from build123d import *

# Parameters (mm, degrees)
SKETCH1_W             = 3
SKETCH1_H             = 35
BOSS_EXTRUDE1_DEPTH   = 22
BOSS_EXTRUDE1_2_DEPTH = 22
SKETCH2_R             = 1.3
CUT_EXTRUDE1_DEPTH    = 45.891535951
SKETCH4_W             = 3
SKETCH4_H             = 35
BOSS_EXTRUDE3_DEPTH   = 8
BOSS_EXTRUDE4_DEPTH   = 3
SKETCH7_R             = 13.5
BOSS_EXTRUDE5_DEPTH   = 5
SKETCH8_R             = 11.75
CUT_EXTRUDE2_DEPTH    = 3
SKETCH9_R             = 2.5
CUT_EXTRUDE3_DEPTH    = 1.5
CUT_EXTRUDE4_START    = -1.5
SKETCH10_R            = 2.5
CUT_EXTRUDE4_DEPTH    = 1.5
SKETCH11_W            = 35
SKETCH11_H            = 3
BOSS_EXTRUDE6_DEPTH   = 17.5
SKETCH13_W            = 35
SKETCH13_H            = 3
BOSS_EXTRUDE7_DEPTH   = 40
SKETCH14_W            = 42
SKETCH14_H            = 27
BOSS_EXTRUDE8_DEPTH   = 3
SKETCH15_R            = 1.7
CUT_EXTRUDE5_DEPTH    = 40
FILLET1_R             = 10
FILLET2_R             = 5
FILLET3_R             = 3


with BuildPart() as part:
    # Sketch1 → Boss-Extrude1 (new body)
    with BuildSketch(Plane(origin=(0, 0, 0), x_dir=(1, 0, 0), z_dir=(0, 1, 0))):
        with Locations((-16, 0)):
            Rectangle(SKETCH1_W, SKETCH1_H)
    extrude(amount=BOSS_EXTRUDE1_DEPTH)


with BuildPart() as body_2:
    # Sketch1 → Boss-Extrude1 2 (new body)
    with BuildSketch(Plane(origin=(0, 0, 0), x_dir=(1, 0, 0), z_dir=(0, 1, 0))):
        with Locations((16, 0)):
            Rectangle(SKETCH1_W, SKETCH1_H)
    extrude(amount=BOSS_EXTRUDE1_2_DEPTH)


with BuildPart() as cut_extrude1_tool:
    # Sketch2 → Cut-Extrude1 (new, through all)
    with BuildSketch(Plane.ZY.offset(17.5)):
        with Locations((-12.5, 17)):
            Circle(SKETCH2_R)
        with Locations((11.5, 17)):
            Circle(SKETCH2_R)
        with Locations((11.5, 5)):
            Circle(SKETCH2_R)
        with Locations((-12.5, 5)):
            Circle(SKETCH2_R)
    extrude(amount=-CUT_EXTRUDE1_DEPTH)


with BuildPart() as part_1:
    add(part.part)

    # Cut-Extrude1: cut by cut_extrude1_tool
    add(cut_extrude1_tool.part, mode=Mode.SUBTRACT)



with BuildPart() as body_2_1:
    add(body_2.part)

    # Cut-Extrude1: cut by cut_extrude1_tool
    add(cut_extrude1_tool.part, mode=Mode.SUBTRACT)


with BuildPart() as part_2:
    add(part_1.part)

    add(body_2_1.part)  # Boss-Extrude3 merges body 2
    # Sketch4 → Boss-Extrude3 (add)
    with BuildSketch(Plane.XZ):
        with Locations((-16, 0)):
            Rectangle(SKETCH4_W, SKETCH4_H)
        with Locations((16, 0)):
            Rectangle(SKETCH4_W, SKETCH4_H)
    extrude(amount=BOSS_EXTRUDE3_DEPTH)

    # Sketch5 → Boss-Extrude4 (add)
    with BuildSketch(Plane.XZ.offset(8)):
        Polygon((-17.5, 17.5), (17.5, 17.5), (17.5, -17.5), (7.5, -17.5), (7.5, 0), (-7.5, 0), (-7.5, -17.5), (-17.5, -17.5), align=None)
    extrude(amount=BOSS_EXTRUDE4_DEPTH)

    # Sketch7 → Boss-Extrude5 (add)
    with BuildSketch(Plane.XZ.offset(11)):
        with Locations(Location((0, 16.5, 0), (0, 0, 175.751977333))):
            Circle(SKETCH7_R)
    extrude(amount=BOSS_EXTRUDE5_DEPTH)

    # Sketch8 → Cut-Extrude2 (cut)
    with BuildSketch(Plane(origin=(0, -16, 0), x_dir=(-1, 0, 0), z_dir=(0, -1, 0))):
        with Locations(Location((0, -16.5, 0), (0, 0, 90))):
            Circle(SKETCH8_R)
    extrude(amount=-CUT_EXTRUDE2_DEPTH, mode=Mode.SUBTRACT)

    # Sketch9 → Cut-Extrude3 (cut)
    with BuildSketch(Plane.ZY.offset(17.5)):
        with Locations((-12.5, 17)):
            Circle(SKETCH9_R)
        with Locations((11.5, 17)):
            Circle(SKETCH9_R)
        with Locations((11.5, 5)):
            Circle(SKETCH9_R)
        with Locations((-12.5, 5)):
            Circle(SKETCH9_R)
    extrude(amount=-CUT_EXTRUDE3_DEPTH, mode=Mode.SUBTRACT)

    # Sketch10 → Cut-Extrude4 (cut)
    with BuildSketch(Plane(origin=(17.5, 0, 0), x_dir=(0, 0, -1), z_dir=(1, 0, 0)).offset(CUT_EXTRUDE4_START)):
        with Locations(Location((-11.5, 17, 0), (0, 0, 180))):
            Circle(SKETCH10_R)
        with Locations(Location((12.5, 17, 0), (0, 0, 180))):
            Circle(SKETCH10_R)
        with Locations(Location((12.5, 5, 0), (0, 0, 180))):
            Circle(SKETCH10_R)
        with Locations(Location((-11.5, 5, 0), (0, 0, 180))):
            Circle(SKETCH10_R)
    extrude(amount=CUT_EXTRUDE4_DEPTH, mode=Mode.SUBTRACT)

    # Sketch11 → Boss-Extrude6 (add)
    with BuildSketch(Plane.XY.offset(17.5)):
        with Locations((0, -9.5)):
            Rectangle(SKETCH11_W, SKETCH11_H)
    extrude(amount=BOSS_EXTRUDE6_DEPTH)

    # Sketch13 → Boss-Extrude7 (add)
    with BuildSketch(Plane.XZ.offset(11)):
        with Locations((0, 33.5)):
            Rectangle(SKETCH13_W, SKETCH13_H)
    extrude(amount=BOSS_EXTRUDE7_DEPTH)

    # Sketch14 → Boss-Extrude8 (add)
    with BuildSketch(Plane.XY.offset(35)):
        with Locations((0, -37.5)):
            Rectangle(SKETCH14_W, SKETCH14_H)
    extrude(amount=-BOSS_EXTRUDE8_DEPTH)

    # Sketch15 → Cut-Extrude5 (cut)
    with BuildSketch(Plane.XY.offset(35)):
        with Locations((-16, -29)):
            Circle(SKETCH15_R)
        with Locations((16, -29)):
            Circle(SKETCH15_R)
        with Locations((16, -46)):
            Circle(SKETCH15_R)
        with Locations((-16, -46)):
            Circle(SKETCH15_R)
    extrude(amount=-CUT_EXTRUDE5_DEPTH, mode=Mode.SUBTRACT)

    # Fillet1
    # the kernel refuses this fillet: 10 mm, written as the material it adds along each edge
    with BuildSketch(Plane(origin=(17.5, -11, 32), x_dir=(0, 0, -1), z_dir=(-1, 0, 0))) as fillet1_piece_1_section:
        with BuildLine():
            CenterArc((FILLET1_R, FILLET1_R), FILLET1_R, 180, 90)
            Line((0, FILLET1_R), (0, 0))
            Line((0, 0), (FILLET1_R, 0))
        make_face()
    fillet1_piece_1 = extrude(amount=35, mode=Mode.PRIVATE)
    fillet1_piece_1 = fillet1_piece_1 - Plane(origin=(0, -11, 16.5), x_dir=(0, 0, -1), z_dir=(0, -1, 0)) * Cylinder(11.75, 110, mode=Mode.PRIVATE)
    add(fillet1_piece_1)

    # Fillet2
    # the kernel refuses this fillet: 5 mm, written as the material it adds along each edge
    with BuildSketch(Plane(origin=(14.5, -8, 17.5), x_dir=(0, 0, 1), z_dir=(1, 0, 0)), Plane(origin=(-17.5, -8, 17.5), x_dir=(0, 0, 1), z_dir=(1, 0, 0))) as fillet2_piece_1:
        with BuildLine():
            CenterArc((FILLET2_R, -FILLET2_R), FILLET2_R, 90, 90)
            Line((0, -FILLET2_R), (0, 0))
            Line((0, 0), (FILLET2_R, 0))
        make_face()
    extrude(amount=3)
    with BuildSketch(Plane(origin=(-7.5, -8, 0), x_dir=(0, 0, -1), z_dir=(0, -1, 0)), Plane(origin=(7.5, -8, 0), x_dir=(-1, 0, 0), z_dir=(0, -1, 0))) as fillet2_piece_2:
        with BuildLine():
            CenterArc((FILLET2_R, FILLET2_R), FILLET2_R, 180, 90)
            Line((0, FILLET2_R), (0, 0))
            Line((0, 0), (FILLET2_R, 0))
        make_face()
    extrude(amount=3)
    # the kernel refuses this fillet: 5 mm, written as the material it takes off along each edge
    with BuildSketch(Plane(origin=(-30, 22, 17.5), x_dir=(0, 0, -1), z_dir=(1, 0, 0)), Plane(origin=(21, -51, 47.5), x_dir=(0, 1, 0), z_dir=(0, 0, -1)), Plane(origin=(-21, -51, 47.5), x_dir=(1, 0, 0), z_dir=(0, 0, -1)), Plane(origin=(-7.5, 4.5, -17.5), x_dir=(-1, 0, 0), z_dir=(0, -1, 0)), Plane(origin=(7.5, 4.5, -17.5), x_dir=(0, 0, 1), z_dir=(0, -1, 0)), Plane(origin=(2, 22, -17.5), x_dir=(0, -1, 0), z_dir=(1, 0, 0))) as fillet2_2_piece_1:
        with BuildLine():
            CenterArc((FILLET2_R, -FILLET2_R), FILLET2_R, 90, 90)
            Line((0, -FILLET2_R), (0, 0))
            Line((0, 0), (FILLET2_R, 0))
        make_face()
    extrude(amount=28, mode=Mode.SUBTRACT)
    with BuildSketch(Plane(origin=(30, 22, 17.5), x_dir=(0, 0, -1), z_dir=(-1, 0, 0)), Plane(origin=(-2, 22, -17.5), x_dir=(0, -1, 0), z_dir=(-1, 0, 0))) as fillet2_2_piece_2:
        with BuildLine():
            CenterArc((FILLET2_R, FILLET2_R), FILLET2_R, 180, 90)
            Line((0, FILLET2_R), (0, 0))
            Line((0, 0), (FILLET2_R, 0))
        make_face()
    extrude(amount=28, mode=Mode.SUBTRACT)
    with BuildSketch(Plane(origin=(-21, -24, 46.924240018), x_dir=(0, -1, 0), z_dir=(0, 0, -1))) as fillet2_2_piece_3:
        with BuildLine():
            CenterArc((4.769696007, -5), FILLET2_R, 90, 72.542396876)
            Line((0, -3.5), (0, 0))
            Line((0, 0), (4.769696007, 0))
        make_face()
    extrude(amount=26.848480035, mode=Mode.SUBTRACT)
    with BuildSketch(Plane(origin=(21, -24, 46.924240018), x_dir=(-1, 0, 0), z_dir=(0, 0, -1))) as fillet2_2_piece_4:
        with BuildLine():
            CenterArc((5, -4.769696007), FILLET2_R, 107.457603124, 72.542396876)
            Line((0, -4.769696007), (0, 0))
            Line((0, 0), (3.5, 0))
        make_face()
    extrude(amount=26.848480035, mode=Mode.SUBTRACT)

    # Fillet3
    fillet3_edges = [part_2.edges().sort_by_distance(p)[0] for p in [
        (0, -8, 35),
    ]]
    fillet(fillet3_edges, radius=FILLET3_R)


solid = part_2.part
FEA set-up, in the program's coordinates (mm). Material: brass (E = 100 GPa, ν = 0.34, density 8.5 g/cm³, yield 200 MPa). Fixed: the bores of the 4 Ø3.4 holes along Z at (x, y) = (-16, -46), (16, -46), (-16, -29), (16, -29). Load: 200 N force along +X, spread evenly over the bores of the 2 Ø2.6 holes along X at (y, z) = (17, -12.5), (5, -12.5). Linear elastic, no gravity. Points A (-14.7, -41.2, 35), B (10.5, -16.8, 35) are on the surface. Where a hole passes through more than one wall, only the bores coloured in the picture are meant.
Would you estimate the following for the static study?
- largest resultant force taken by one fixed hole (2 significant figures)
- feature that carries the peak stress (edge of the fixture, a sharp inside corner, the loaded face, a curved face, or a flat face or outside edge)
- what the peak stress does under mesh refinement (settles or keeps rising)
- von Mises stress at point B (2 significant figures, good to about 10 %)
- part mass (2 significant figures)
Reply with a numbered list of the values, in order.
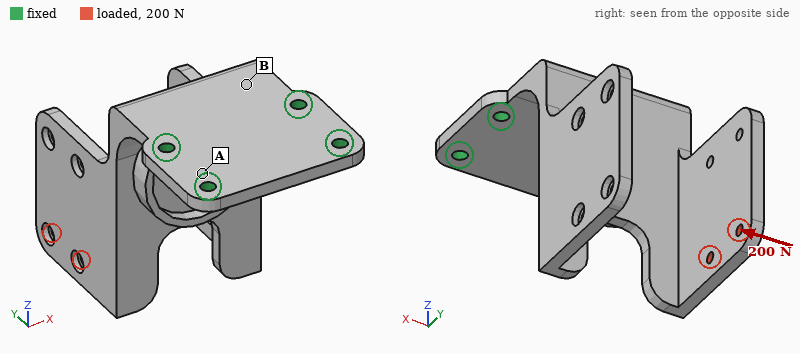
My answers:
1. 410 N
2. edge of the fixture
3. keeps rising
4. 38 MPa
5. 150 g
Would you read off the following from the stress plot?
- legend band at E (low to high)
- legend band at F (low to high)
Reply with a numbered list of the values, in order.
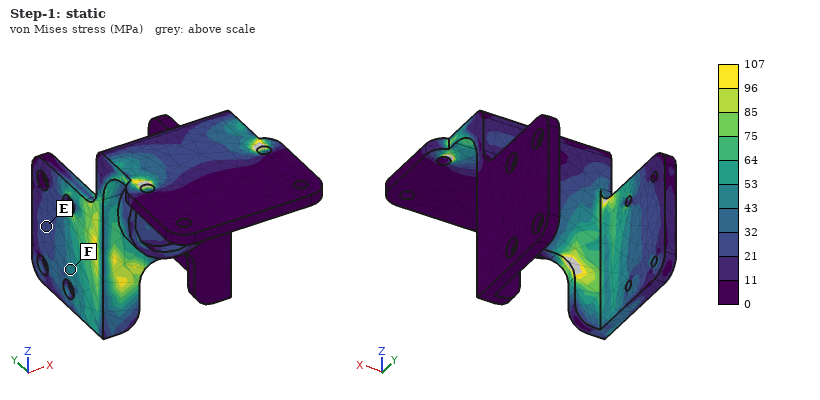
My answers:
1. 21 to 32 MPa
2. 43 to 53 MPa
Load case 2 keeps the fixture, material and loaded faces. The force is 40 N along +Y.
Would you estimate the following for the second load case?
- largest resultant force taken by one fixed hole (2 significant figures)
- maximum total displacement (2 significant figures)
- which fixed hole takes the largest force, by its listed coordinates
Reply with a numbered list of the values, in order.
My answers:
1. 37 N
2. 0.24 mm
3. (-16, -29)
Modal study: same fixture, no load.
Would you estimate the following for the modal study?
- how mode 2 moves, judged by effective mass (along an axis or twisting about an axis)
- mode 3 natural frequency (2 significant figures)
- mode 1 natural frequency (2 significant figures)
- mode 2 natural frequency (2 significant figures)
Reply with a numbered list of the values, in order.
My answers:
1. along X
2. 1000 Hz
3. 310 Hz
4. 820 Hz
